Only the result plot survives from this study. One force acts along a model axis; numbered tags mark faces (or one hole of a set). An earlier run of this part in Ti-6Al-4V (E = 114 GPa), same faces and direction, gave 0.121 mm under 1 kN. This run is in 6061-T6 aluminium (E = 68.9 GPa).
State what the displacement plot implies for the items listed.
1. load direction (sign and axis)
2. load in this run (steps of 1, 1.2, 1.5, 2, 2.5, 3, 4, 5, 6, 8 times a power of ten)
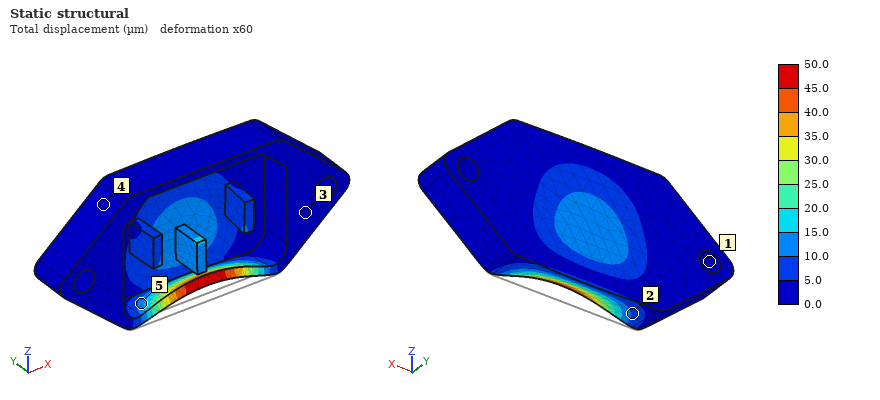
+Z
250 N
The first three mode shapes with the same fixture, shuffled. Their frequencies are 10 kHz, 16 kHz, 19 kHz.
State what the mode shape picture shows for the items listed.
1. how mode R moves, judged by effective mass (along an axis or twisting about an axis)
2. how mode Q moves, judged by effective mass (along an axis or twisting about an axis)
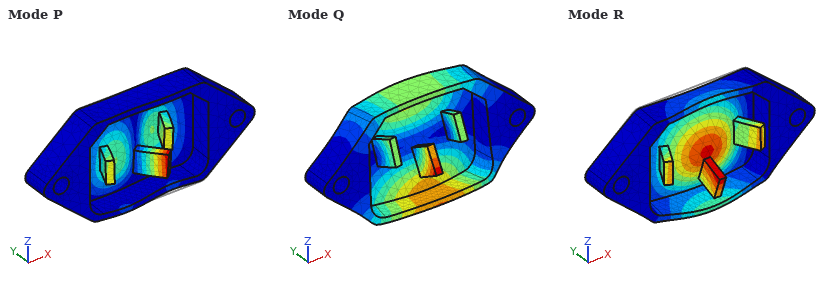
along Y
twisting about X
